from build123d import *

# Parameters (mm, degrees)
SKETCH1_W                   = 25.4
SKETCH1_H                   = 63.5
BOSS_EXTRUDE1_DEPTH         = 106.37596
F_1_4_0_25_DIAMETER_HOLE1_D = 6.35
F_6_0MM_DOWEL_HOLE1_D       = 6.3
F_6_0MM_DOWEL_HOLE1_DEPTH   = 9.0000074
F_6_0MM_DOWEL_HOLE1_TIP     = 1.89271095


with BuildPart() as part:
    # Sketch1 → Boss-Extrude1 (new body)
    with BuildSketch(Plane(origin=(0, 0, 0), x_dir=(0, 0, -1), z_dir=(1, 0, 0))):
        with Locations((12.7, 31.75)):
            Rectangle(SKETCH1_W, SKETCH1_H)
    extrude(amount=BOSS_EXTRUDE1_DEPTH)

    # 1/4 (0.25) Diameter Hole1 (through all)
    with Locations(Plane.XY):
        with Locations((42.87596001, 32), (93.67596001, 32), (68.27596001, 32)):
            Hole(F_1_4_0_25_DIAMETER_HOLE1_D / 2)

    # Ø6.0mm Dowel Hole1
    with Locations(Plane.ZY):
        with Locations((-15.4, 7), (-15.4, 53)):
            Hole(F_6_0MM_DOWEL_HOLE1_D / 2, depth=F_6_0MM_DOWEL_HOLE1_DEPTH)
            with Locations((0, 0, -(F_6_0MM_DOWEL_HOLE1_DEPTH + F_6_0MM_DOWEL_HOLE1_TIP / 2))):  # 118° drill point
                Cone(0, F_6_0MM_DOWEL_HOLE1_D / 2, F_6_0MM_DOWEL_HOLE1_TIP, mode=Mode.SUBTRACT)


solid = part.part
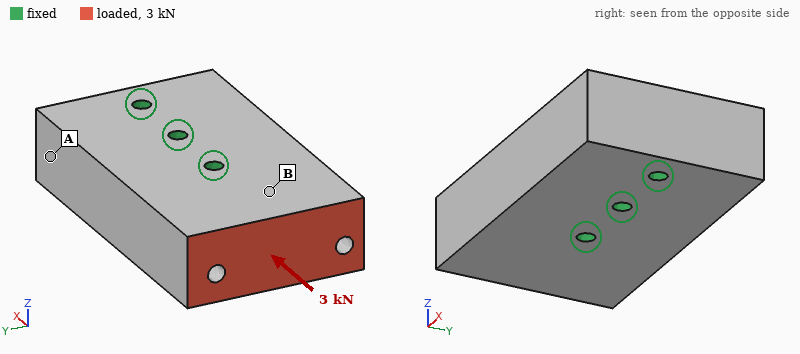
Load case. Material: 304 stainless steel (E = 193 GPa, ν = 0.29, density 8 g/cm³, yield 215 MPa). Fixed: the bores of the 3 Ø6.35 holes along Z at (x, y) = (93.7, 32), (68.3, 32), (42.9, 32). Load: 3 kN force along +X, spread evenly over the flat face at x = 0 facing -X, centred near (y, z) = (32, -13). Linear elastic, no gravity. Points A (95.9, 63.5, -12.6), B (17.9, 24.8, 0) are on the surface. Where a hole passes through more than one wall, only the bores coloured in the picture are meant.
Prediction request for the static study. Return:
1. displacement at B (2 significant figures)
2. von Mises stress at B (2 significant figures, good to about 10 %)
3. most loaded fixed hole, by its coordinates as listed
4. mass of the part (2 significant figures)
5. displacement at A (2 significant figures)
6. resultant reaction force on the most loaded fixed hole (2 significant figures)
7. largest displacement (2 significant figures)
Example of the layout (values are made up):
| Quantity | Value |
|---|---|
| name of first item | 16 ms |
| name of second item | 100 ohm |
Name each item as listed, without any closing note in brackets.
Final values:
| Quantity | Value |
|---|---|
| displacement at B | 0.39 µm |
| von Mises stress at B | 2.3 MPa |
| most loaded fixed hole, by its coordinates as listed | (42.9, 32) |
| mass of the part | 1.3 kg |
| displacement at A | 0.10 µm |
| resultant reaction force on the most loaded fixed hole | 1.9 kN |
| largest displacement | 0.64 µm |
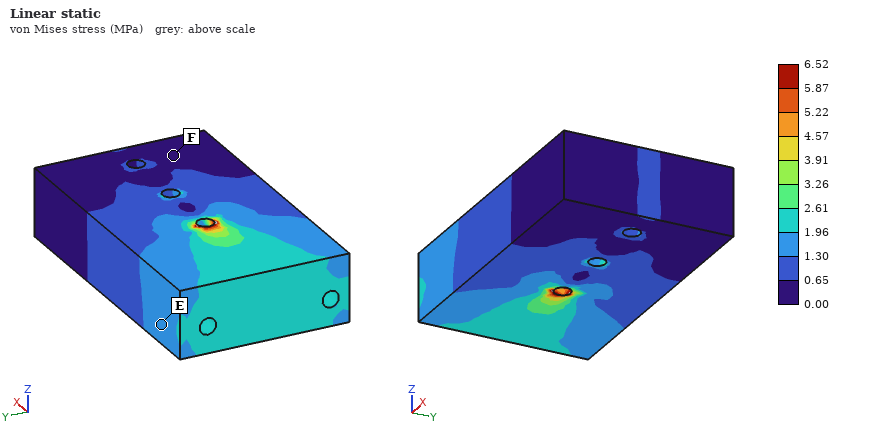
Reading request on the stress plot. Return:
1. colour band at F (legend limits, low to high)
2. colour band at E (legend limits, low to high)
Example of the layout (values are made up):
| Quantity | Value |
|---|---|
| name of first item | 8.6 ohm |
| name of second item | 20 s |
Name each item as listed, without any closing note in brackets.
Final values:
| Quantity | Value |
|---|---|
| colour band at F | 0.00 to 0.65 MPa |
| colour band at E | 1.30 to 1.96 MPa |
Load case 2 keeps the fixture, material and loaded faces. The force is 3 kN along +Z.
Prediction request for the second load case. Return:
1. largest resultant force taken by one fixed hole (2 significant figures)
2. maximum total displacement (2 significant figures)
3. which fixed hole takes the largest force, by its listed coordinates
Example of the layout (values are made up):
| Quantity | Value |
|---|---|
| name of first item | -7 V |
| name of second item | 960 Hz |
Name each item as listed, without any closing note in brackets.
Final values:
| Quantity | Value |
|---|---|
| largest resultant force taken by one fixed hole | 4.3 kN |
| maximum total displacement | 9.4 µm |
| which fixed hole takes the largest force, by its listed coordinates | (42.9, 32) |
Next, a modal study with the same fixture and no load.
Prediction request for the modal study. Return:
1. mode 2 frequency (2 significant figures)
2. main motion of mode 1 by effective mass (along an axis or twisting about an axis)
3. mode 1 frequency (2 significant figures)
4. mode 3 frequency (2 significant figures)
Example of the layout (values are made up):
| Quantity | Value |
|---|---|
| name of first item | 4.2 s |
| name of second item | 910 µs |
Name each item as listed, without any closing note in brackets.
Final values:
| Quantity | Value |
|---|---|
| mode 2 frequency | 8500 Hz |
| main motion of mode 1 by effective mass | along Z |
| mode 1 frequency | 6900 Hz |
| mode 3 frequency | 8700 Hz |
